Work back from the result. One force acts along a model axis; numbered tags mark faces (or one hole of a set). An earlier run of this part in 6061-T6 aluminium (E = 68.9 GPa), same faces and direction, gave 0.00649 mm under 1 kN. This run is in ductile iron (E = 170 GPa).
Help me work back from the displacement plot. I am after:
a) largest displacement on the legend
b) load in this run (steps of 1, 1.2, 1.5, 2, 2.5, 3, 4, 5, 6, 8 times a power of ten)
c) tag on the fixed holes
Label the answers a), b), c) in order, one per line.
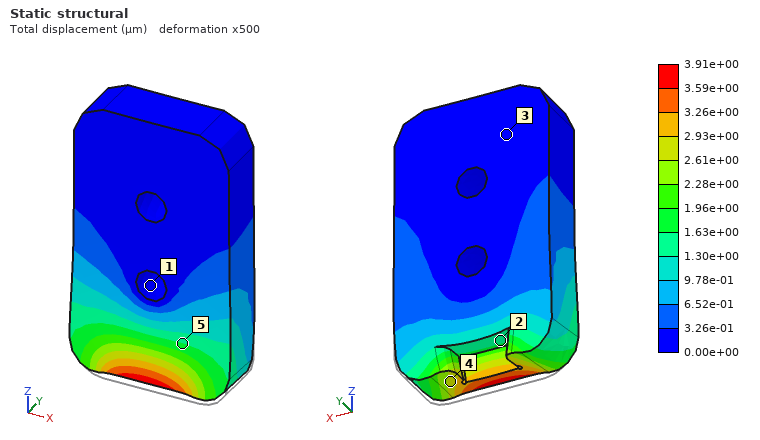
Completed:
a) 3.91e+00 µm
b) 1.5 kN
c) 1
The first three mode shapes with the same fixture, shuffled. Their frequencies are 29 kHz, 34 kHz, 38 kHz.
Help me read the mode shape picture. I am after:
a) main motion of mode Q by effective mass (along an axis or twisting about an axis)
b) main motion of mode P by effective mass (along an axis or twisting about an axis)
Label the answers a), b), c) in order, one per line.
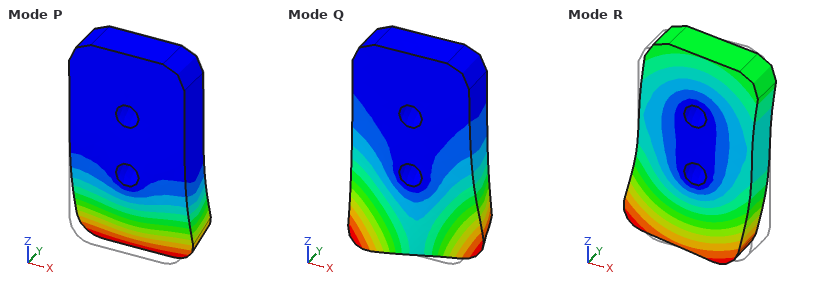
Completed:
a) twisting about Z
b) along Y
